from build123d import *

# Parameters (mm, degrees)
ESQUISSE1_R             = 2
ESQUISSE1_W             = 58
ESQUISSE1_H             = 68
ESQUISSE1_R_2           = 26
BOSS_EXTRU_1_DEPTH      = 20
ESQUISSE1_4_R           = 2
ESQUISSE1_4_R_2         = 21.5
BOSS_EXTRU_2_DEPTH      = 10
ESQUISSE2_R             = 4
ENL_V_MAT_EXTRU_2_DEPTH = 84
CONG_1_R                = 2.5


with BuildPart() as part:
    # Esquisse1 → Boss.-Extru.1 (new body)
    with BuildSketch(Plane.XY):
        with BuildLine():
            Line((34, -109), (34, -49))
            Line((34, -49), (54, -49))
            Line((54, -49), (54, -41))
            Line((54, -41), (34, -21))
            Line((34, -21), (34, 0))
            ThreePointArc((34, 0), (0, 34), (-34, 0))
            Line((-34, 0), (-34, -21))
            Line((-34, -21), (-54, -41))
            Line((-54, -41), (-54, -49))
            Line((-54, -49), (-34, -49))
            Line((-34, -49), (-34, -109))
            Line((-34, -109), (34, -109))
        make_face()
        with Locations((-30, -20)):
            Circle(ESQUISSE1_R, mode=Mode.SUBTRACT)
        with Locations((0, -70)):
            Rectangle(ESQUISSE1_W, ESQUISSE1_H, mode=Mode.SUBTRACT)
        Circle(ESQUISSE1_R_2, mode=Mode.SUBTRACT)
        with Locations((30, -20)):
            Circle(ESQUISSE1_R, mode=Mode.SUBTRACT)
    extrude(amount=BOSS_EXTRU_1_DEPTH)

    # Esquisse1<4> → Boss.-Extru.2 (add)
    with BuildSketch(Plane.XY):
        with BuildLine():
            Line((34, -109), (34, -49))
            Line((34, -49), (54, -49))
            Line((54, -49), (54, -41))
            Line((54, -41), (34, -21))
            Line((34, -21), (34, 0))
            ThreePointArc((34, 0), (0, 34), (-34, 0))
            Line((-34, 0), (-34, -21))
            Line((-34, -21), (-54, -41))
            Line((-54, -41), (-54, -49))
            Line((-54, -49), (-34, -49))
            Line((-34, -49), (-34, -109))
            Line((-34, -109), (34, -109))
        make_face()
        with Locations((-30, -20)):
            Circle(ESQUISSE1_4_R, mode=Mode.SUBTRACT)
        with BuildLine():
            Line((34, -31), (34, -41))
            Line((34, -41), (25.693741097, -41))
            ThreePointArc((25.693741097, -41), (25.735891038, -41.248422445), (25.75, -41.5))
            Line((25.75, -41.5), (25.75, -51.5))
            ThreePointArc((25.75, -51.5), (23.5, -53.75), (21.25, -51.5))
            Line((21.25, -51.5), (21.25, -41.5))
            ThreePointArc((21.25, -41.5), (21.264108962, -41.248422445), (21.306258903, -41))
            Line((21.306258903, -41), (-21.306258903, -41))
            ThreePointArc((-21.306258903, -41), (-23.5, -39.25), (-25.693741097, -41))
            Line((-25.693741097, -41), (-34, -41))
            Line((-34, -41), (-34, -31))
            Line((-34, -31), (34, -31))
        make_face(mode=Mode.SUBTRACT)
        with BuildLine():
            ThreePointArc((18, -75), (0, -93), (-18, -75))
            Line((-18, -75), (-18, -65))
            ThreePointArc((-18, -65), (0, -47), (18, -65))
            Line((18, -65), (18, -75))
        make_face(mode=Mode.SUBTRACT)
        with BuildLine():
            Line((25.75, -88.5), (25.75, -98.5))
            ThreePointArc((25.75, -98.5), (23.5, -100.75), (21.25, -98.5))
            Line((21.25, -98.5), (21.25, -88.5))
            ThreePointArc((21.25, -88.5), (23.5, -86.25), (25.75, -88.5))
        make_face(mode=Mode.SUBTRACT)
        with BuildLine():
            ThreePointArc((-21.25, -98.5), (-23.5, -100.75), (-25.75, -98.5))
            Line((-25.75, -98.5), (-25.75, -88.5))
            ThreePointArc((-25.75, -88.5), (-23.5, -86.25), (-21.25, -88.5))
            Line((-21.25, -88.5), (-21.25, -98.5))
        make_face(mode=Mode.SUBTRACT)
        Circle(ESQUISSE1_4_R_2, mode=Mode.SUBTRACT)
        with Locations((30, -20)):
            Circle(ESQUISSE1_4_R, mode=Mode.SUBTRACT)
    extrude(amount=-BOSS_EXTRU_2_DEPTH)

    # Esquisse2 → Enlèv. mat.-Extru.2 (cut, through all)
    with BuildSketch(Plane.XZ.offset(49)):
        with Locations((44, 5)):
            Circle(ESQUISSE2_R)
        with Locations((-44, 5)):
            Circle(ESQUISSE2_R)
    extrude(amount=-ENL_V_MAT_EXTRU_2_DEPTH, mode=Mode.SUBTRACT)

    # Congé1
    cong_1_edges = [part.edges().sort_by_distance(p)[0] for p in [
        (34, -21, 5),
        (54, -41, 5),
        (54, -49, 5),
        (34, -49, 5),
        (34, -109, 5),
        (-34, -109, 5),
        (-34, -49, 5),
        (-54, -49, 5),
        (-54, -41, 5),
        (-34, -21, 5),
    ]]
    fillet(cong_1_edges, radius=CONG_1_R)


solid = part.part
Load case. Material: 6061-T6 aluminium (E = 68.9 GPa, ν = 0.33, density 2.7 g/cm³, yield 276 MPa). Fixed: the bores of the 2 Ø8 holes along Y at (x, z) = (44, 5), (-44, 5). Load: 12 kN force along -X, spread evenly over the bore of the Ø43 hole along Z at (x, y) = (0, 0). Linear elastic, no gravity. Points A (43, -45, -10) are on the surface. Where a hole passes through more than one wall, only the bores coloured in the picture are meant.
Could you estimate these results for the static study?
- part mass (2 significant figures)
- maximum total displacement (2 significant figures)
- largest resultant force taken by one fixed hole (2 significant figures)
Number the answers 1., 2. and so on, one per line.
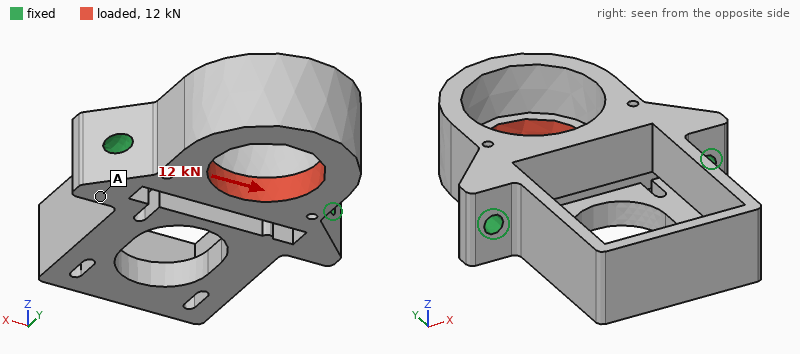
1. 370 g
2. 0.13 mm
3. 7.8 kN
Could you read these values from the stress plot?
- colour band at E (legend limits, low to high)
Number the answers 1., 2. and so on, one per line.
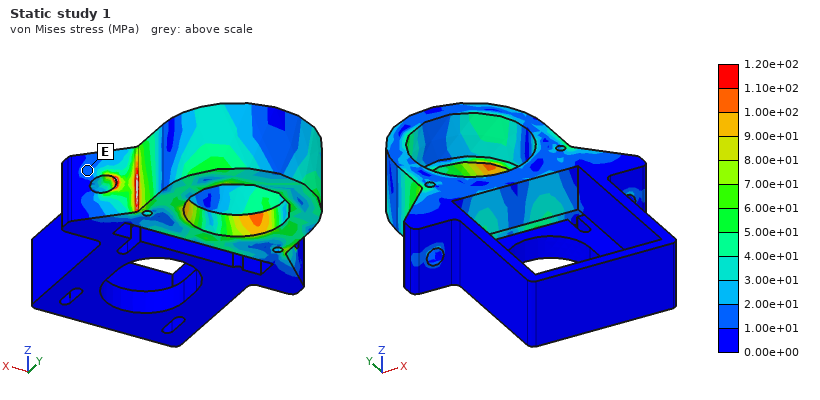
1. 1.00e+01 to 2.00e+01 MPa
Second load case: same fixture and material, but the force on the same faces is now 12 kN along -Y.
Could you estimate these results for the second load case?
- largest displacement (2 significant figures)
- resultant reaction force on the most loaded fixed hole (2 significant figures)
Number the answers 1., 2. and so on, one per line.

1. 0.14 mm
2. 6.7 kN
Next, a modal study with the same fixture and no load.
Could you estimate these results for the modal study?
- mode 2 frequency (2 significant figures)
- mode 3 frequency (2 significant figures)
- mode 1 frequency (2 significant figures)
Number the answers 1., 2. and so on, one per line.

1. 2800 Hz
2. 2900 Hz
3. 2200 Hz
